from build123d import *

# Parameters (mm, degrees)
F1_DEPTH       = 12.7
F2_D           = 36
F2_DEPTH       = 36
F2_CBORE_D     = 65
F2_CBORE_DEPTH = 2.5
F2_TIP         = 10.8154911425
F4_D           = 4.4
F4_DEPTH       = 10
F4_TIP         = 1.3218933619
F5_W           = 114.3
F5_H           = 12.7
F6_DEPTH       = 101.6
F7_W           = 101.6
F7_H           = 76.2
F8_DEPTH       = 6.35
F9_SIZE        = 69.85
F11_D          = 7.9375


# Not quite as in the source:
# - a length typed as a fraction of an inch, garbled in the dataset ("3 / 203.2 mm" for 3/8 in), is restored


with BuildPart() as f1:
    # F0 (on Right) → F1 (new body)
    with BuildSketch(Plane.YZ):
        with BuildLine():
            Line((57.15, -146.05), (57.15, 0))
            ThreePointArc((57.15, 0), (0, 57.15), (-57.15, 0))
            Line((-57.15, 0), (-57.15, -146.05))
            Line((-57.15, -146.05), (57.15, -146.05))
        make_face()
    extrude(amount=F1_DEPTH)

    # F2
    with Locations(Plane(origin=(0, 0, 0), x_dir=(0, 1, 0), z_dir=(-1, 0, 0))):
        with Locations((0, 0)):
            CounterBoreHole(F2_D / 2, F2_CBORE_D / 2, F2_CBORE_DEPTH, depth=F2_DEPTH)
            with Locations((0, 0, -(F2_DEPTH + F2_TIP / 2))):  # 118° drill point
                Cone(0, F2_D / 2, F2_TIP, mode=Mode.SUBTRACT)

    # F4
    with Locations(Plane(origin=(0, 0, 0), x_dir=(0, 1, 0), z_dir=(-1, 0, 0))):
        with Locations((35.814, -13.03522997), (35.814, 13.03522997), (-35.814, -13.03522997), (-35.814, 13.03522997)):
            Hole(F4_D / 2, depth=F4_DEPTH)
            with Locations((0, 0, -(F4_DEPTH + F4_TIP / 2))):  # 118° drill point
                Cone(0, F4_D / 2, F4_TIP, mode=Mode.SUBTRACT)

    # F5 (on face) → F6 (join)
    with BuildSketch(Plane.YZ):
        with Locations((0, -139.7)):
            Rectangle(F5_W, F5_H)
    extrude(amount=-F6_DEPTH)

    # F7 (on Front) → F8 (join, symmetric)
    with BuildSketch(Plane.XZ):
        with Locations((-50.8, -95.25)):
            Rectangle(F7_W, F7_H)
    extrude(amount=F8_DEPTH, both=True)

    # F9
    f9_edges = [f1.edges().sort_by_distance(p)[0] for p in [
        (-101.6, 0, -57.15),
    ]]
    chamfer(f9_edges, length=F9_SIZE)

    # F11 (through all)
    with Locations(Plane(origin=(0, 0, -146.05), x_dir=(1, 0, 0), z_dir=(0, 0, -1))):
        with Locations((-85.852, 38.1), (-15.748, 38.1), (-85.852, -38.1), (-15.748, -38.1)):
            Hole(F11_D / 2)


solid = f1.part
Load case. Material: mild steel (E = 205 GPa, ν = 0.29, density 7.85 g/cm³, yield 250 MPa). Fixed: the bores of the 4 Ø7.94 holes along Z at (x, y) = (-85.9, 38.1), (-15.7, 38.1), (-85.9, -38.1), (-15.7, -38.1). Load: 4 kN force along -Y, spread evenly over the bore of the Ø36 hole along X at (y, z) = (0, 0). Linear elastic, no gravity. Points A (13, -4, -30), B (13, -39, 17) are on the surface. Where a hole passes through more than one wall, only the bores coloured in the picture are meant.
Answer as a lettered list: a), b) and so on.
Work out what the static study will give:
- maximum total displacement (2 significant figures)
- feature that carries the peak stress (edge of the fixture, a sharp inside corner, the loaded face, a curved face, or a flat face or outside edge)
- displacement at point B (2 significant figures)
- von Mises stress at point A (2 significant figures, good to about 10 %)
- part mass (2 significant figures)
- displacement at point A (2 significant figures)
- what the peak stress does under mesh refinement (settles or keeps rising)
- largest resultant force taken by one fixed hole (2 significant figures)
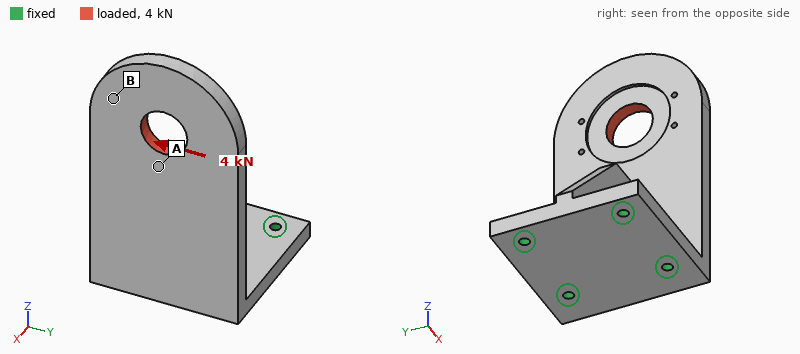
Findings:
a) 83 µm
b) edge of the fixture
c) 67 µm
d) 11 MPa
e) 3.7 kg
f) 43 µm
g) keeps rising
h) 7.3 kN
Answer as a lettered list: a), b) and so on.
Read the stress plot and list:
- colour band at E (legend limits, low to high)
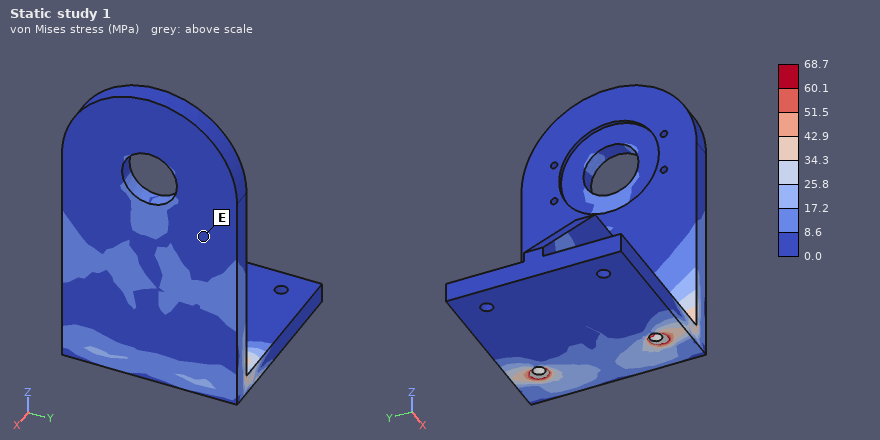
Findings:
a) 0.0 to 8.6 MPa
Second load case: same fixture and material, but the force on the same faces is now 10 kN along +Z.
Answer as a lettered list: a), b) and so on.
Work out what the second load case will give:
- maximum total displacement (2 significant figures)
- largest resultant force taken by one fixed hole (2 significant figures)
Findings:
a) 57 µm
b) 6.0 kN
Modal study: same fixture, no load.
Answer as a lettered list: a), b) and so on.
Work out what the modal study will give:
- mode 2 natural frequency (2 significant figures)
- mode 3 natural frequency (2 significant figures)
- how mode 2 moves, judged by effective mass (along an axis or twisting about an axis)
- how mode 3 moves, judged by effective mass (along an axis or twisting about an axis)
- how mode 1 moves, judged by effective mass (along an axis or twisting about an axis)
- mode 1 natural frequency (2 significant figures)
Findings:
a) 1100 Hz
b) 1300 Hz
c) along Y
d) along Y
e) along X
f) 650 Hz
